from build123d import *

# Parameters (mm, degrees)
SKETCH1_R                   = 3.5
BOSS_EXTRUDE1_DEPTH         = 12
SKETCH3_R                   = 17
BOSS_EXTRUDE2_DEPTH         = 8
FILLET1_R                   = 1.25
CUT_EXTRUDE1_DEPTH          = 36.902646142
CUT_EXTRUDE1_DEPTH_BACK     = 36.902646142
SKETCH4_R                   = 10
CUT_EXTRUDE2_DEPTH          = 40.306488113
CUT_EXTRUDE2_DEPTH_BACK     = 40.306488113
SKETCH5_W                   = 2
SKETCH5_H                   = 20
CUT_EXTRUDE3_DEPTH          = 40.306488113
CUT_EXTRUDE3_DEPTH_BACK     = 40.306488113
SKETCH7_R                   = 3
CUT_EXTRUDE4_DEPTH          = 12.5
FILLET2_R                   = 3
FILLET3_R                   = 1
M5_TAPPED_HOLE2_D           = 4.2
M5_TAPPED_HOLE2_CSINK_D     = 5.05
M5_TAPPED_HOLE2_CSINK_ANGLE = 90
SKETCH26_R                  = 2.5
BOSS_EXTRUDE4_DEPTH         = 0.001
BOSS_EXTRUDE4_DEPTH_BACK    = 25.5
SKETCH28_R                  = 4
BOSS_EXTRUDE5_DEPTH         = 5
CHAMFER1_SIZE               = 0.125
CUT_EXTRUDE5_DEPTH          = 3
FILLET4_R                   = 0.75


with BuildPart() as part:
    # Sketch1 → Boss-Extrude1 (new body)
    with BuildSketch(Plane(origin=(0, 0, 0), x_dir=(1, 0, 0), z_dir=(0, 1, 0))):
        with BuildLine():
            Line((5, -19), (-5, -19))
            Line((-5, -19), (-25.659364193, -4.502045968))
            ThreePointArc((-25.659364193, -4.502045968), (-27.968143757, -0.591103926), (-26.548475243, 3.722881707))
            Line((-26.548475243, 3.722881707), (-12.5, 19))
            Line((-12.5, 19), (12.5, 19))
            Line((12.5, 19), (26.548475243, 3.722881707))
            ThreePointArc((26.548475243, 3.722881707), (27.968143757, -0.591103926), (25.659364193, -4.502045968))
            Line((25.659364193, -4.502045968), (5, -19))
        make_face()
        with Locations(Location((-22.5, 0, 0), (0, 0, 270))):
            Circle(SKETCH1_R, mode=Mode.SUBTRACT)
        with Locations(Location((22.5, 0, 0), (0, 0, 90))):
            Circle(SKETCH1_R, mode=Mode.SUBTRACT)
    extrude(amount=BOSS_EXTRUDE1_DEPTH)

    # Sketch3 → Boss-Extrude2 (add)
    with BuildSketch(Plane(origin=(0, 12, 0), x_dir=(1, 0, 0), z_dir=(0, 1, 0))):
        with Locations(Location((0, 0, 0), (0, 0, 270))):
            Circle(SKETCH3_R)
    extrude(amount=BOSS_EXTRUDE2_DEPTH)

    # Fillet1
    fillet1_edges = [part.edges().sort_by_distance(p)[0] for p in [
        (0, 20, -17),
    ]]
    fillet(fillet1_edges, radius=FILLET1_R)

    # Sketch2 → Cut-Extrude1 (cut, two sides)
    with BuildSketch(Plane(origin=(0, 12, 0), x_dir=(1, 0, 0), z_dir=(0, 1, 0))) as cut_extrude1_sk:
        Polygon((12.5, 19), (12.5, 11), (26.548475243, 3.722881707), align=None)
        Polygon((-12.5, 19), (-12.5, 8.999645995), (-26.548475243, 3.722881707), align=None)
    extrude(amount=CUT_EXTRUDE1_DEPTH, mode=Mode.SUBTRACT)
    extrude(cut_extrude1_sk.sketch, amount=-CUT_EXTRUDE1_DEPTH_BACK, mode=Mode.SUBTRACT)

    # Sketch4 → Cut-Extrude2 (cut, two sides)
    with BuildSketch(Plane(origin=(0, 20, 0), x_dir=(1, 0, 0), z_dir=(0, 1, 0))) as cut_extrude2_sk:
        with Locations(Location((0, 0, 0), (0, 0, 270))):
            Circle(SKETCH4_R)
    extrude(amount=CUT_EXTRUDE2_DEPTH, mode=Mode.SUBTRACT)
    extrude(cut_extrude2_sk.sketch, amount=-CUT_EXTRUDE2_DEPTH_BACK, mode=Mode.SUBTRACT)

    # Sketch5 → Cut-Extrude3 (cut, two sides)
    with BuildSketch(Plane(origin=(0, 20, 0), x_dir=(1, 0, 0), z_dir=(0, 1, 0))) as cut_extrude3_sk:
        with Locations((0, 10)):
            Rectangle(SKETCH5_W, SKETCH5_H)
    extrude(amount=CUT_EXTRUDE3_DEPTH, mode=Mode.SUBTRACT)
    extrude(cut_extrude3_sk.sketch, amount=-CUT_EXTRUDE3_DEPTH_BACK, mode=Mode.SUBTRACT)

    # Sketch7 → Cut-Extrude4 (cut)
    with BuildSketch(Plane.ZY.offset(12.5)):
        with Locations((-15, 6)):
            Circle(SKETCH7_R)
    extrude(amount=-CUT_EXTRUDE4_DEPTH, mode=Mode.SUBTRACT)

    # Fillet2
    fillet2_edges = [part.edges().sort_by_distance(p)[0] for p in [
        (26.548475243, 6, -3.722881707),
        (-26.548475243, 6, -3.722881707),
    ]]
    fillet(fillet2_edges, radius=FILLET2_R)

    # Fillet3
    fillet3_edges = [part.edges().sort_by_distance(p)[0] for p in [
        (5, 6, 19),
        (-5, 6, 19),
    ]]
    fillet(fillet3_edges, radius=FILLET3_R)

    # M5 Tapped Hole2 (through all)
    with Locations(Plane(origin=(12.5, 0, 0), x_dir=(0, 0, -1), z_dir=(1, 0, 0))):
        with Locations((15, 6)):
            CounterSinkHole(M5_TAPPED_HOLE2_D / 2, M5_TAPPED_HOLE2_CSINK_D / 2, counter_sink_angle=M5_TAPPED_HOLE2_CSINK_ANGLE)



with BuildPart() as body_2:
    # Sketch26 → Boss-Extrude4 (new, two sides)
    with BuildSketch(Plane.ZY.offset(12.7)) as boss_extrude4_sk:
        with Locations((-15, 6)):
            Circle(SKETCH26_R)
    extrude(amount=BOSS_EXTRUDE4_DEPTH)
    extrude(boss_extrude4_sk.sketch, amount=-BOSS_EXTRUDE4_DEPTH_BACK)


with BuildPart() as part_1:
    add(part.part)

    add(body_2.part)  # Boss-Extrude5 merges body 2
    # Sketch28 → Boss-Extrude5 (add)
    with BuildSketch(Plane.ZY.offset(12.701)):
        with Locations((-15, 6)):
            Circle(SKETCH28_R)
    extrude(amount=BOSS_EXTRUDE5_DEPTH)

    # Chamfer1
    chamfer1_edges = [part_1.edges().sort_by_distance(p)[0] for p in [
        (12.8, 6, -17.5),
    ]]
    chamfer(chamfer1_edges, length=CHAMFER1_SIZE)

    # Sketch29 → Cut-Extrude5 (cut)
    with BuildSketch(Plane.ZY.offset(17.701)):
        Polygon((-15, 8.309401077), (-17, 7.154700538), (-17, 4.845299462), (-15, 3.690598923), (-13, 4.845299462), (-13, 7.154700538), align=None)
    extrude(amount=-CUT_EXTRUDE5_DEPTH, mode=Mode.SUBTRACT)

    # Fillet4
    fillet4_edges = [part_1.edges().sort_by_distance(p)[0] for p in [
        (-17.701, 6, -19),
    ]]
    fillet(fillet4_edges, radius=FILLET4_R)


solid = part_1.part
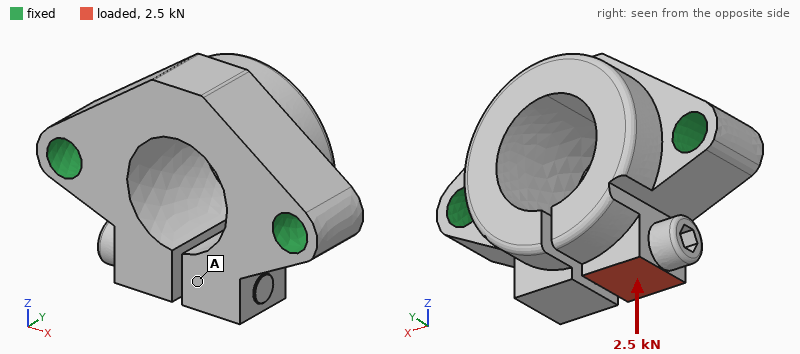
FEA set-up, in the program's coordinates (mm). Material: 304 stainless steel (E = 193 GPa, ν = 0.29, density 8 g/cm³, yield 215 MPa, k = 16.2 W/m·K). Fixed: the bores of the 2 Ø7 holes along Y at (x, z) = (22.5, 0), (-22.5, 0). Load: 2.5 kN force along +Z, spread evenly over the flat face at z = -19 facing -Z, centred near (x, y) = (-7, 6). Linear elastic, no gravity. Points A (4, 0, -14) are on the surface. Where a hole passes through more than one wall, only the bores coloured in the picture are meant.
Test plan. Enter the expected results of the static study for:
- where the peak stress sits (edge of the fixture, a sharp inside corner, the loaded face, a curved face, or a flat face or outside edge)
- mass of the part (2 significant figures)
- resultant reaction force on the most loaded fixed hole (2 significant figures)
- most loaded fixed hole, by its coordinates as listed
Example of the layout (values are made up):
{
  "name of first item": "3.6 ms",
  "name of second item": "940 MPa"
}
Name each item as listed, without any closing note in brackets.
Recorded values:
{
  "where the peak stress sits": "a curved face",
  "mass of the part": "130 g",
  "resultant reaction force on the most loaded fixed hole": "2.3 kN",
  "most loaded fixed hole, by its coordinates as listed": "(-22.5, 0)"
}
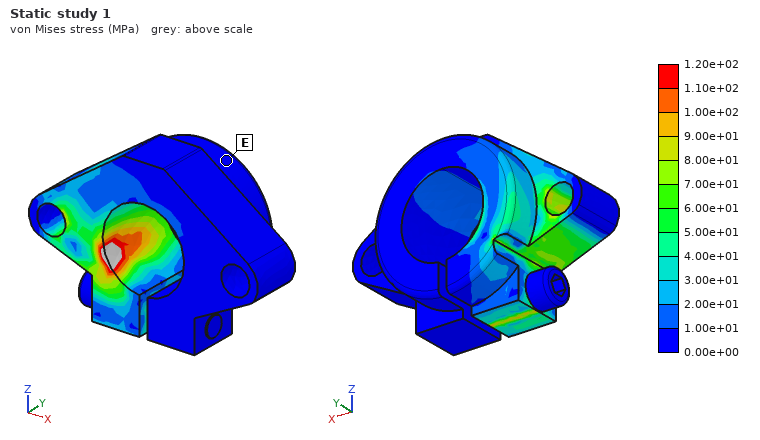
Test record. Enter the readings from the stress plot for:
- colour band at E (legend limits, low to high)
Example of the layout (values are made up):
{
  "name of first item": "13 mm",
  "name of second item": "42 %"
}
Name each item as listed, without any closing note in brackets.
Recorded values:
{
  "colour band at E": "0.00e+00 to 1.00e+01 MPa"
}
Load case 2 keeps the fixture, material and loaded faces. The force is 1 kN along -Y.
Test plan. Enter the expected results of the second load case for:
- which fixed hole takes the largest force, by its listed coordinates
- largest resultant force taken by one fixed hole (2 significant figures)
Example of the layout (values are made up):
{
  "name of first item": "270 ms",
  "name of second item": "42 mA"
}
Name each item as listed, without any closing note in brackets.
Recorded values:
{
  "which fixed hole takes the largest force, by its listed coordinates": "(-22.5, 0)",
  "largest resultant force taken by one fixed hole": "1.0 kN"
}
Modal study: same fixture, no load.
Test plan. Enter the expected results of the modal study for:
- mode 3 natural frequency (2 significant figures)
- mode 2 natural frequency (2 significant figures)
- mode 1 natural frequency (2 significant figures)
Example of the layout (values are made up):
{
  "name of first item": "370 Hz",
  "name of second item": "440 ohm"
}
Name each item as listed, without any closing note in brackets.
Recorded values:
{
  "mode 3 natural frequency": "11 kHz",
  "mode 2 natural frequency": "5800 Hz",
  "mode 1 natural frequency": "5400 Hz"
}
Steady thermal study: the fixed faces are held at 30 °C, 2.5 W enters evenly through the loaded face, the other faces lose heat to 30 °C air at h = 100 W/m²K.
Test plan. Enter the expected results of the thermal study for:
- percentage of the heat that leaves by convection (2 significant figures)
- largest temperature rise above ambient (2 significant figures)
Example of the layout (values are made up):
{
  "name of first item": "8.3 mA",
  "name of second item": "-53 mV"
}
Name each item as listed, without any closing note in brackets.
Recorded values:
{
  "percentage of the heat that leaves by convection": "59 %",
  "largest temperature rise above ambient": "23 K"
}
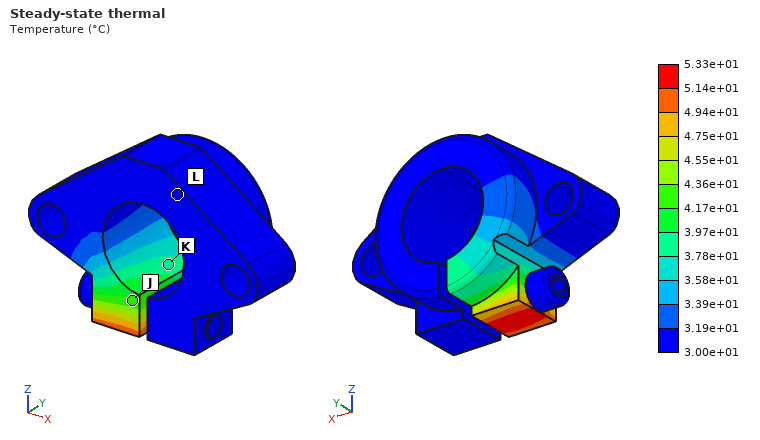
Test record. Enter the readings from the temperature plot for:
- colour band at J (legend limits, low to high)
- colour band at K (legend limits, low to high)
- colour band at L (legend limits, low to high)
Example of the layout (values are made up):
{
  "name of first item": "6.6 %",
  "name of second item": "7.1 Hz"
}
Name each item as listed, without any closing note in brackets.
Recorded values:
{
  "colour band at J": "4.17e+01 to 4.36e+01 °C",
  "colour band at K": "3.78e+01 to 3.97e+01 °C",
  "colour band at L": "3.00e+01 to 3.19e+01 °C"
}
